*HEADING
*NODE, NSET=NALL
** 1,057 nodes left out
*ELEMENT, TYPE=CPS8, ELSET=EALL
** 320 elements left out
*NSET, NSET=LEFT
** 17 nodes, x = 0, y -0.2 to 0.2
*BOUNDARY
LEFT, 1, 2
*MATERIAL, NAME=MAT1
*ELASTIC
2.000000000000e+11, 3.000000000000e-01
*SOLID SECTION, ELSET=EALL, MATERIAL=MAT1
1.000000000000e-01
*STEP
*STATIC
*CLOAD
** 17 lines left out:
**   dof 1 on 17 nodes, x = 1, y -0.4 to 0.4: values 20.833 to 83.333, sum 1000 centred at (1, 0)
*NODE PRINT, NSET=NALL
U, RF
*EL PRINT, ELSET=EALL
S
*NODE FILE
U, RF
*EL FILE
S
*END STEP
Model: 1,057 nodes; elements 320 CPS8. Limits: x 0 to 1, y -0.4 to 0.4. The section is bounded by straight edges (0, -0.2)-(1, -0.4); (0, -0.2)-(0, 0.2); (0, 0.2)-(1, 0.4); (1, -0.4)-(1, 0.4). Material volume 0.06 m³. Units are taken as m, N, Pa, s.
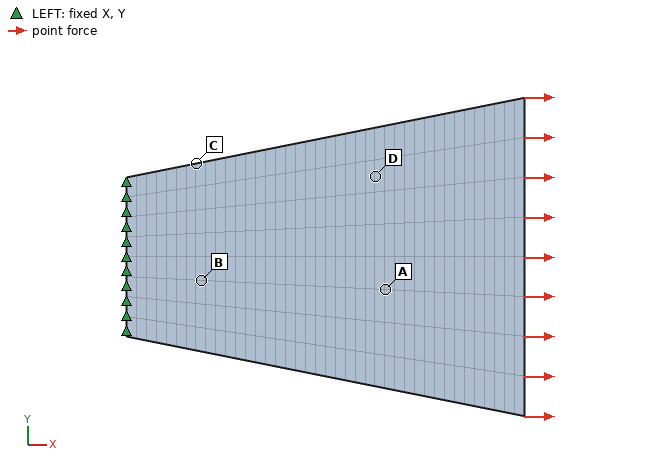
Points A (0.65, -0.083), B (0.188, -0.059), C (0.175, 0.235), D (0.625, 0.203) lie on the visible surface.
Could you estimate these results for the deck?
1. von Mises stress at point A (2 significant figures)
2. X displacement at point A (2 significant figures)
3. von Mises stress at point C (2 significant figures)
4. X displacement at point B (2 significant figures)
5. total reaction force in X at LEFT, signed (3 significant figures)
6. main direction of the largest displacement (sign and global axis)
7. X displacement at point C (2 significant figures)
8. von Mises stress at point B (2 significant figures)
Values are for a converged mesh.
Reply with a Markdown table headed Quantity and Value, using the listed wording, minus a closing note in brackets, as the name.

| Quantity | Value |
|---|---|
| von Mises stress at point A | 15000 Pa |
| X displacement at point A | 6.1e-08 m |
| von Mises stress at point C | 20000 Pa |
| X displacement at point B | 2.0e-08 m |
| total reaction force in X at LEFT, signed | -1000 N |
| main direction of the largest displacement | +X |
| X displacement at point C | 2.4e-08 m |
| von Mises stress at point B | 21000 Pa |
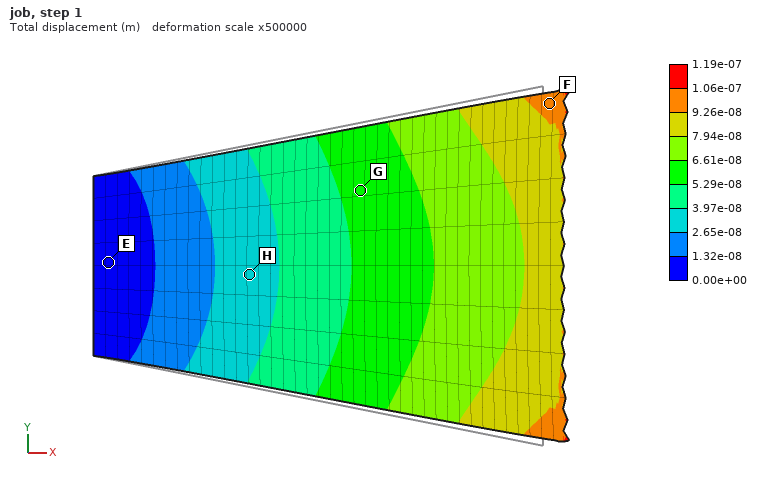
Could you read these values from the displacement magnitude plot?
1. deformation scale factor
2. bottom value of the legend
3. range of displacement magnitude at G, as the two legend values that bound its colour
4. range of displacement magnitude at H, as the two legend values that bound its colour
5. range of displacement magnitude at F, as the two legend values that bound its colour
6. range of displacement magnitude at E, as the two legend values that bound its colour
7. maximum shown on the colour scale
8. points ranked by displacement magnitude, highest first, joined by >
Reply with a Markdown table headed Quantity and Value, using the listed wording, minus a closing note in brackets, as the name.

| Quantity | Value |
|---|---|
| deformation scale factor | 500000 |
| bottom value of the legend | 0.00e+00 m |
| range of displacement magnitude at G, as the two legend values that bound its colour | 5.29e-08 to 6.61e-08 m |
| range of displacement magnitude at H, as the two legend values that bound its colour | 2.65e-08 to 3.97e-08 m |
| range of displacement magnitude at F, as the two legend values that bound its colour | 9.26e-08 to 1.06e-07 m |
| range of displacement magnitude at E, as the two legend values that bound its colour | 0.00e+00 to 1.32e-08 m |
| maximum shown on the colour scale | 1.19e-07 m |
| points ranked by displacement magnitude, highest first, joined by > | F > G > H > E |
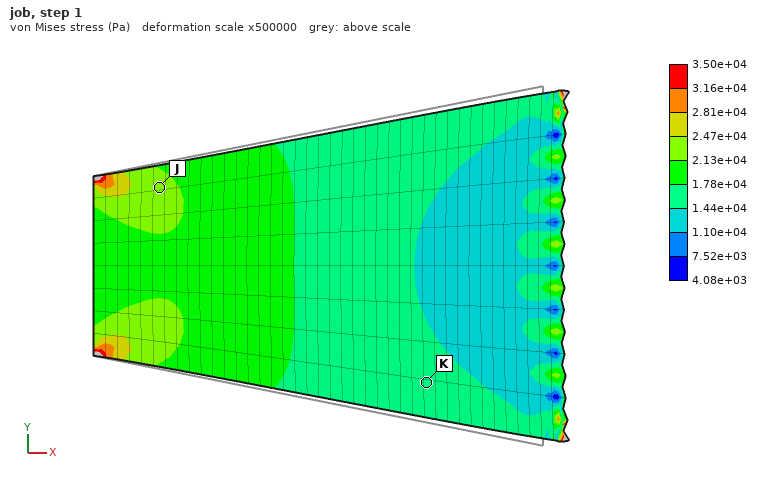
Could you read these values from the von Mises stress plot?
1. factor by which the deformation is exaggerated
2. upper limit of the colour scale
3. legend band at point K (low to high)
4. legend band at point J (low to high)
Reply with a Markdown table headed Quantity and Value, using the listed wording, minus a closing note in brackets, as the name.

| Quantity | Value |
|---|---|
| factor by which the deformation is exaggerated | 500000 |
| upper limit of the colour scale | 3.50e+04 Pa |
| legend band at point K | 1.44e+04 to 1.78e+04 Pa |
| legend band at point J | 2.13e+04 to 2.47e+04 Pa |
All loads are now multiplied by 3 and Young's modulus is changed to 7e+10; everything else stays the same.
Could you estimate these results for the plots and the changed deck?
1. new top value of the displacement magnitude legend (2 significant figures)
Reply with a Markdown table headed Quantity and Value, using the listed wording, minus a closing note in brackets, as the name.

| Quantity | Value |
|---|---|
| new top value of the displacement magnitude legend | 1.0e-06 m |
